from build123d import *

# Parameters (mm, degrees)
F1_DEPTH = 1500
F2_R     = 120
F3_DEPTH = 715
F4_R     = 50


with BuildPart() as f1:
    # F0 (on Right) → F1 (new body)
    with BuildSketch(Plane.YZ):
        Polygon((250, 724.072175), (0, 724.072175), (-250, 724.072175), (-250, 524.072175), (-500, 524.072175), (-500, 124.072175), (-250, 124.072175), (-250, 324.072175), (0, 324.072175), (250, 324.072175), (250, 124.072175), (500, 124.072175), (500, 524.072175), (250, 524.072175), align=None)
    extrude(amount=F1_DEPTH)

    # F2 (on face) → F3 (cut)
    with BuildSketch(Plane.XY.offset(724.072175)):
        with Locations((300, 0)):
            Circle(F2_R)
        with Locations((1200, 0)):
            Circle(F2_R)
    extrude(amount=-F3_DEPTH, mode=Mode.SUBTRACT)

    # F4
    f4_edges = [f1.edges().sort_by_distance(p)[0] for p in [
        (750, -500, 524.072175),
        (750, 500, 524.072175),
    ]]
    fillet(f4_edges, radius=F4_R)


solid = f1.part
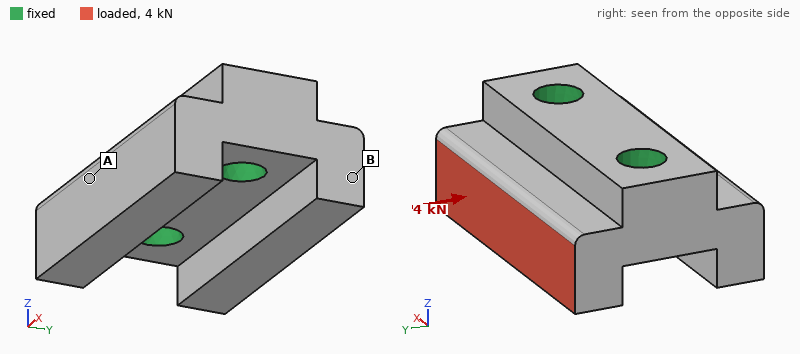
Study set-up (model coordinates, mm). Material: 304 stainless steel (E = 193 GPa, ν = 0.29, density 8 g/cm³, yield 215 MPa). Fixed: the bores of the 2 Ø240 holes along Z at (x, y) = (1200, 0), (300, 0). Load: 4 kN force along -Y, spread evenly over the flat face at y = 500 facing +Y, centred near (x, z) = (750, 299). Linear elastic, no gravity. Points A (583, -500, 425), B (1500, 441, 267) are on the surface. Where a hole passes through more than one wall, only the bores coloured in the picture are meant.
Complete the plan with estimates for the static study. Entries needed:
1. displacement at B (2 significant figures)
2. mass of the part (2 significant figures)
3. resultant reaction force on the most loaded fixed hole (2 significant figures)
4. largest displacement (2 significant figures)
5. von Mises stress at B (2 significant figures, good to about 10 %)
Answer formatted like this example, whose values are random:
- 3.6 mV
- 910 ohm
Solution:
- 0.15 µm
- 4500 kg
- 2.0 kN
- 0.25 µm
- 0.012 MPa
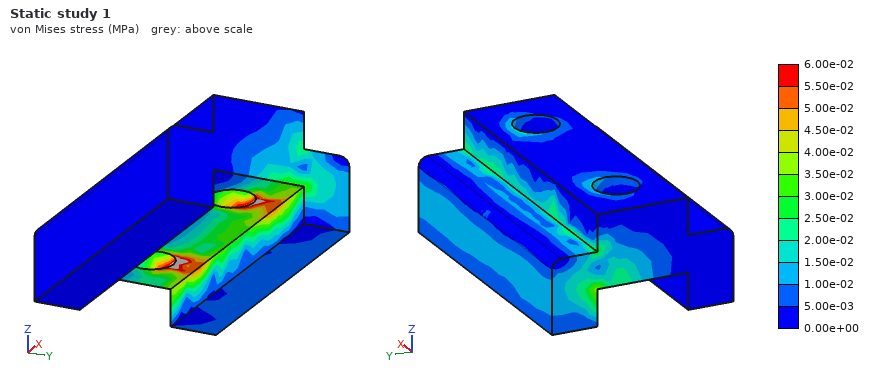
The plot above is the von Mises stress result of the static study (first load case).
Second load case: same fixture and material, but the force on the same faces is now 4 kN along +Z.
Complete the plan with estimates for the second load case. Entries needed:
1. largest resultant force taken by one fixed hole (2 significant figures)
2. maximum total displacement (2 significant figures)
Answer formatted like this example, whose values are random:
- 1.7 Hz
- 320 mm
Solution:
- 2.0 kN
- 0.51 µm
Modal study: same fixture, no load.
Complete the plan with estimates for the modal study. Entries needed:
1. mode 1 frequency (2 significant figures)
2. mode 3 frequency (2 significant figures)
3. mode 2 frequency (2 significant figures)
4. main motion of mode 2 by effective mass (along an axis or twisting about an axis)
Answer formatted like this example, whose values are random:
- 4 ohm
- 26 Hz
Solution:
- 570 Hz
- 770 Hz
- 630 Hz
- along Z
